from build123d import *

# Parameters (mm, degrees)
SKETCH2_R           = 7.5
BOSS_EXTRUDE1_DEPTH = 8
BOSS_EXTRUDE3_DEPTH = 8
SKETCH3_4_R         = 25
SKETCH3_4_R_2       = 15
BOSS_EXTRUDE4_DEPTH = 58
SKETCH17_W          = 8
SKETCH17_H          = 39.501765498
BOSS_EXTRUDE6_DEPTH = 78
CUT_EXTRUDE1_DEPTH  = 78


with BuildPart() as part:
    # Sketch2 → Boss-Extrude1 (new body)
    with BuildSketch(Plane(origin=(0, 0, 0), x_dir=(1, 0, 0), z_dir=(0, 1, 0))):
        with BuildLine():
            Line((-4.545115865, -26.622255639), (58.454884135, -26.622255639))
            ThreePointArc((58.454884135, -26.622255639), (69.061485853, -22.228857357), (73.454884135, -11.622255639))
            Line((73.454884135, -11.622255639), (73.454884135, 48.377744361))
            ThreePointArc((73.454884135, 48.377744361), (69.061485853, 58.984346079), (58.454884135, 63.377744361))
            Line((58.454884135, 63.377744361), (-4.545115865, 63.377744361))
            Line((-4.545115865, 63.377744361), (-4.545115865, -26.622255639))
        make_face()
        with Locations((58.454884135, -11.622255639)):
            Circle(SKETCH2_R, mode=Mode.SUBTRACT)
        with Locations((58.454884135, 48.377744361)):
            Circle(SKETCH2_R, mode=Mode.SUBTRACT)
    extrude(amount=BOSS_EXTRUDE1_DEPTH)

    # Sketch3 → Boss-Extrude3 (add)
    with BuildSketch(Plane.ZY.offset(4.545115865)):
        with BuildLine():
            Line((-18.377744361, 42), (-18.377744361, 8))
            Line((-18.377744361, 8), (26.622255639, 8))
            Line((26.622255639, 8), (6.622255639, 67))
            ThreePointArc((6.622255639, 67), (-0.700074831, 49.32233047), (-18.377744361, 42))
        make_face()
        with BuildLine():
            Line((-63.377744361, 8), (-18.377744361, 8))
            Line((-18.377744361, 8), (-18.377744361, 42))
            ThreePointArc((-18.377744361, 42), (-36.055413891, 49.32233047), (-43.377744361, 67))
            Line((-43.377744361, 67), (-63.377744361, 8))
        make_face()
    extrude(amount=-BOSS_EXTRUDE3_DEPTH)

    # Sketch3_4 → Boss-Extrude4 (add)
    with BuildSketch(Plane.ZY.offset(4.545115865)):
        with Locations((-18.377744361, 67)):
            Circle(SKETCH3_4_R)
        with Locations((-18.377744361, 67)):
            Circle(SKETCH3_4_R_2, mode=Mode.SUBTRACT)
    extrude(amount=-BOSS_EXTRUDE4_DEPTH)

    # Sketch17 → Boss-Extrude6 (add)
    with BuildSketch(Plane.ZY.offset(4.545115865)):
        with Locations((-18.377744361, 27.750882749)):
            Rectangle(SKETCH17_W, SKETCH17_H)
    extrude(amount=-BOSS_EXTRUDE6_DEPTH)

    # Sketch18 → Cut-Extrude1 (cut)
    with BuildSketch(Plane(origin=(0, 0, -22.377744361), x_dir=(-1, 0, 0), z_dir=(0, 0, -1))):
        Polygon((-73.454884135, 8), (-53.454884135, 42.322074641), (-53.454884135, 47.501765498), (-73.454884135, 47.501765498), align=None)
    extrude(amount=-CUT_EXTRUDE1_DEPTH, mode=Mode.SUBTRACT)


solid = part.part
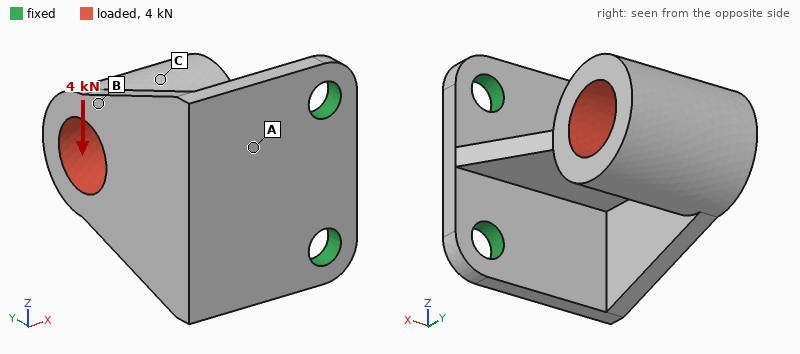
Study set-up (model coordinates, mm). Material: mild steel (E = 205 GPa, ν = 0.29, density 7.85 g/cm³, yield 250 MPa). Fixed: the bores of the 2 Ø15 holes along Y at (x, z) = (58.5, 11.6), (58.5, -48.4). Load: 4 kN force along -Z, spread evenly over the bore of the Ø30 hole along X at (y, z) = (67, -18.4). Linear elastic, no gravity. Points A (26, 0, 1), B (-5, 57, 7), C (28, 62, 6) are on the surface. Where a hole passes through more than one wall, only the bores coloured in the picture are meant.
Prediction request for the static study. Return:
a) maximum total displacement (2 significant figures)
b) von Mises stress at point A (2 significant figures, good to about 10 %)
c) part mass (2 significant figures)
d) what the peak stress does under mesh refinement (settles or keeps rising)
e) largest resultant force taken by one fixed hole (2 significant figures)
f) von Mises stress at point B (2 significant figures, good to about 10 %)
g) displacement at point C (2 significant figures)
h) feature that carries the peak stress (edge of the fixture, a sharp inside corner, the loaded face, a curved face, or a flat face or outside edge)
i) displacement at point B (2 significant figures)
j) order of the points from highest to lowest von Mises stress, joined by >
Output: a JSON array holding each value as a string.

["0.30 mm", "87 MPa", "1.3 kg", "keeps rising", "5.5 kN", "43 MPa", "0.22 mm", "edge of the fixture", "0.20 mm", "A > B > C"]
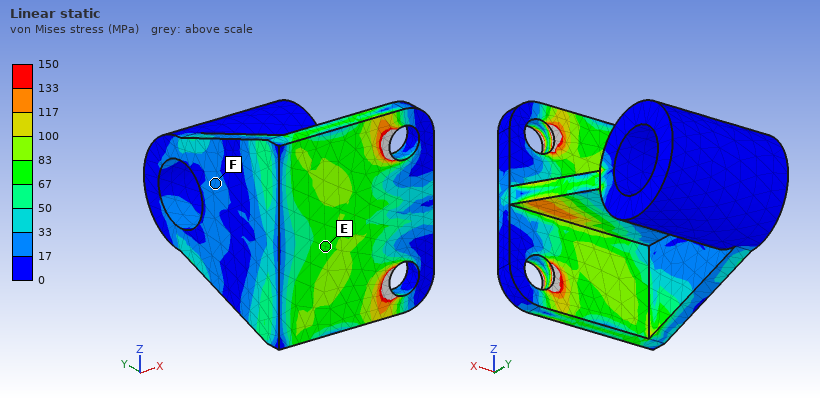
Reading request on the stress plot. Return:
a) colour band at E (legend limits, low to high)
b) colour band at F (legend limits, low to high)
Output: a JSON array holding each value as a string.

["67 to 83 MPa", "17 to 33 MPa"]
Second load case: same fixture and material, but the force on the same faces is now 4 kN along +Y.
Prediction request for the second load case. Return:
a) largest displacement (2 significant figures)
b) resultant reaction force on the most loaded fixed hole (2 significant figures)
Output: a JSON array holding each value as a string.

["0.15 mm", "2.0 kN"]
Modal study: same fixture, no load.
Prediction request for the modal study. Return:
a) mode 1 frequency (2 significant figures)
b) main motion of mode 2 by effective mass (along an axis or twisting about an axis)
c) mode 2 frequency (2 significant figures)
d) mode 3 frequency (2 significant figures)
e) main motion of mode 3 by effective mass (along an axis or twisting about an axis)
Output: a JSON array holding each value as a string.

["690 Hz", "along Z", "800 Hz", "2900 Hz", "twisting about Y"]
